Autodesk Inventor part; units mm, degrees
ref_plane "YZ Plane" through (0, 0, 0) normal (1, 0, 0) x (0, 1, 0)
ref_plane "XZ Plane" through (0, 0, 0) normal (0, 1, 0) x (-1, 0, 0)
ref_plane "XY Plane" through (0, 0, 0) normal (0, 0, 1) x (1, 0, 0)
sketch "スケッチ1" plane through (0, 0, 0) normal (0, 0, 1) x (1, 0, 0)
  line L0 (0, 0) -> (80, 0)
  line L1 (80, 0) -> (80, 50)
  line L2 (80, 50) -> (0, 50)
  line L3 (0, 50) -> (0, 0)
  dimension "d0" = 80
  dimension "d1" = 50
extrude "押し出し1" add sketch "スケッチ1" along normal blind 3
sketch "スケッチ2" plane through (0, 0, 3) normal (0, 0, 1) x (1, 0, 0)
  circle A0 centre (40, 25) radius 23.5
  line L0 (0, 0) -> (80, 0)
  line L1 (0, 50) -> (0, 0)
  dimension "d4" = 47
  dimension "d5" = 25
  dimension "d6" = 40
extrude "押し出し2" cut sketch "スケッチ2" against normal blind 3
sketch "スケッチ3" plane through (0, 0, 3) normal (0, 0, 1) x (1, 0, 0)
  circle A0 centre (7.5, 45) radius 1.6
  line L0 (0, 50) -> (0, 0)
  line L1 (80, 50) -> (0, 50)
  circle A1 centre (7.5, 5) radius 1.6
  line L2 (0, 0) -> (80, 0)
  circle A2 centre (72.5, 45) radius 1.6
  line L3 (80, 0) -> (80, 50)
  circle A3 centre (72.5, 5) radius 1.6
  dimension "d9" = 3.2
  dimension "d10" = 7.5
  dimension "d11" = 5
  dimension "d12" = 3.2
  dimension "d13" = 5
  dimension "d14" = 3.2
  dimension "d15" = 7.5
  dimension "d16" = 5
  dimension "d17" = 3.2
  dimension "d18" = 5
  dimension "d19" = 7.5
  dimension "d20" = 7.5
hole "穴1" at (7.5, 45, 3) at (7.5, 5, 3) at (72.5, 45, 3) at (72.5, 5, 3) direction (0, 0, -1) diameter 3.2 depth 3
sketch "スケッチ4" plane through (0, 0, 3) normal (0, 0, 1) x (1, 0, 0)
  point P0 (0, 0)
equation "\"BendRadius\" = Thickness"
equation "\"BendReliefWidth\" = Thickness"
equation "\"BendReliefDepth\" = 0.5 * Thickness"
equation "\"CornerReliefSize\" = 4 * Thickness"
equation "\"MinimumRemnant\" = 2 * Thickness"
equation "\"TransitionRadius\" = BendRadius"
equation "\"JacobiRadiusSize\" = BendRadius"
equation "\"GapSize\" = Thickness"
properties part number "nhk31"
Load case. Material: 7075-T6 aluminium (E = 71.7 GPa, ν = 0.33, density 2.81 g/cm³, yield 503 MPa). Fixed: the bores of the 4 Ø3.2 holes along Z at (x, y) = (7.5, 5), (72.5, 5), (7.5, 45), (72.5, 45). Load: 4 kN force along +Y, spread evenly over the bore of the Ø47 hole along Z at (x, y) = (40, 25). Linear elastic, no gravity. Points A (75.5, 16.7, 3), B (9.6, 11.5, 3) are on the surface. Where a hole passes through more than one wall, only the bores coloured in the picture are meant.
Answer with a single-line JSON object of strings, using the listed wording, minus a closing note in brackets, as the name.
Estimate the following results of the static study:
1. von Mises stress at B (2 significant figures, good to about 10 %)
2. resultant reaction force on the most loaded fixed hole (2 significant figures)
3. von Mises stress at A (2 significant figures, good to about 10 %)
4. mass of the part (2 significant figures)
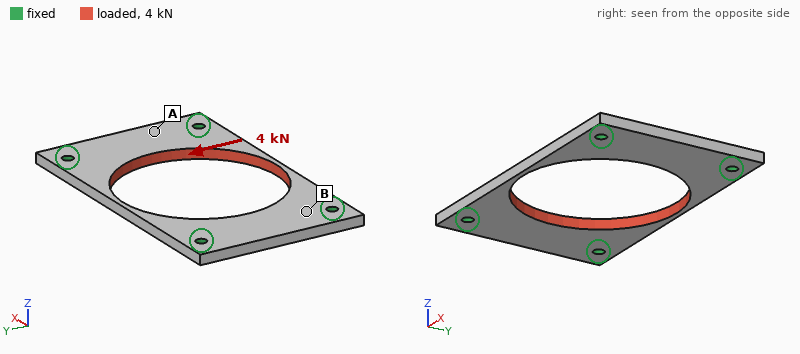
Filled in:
{"von Mises stress at B": "34 MPa", "resultant reaction force on the most loaded fixed hole": "1.0 kN", "von Mises stress at A": "20 MPa", "mass of the part": "19 g"}
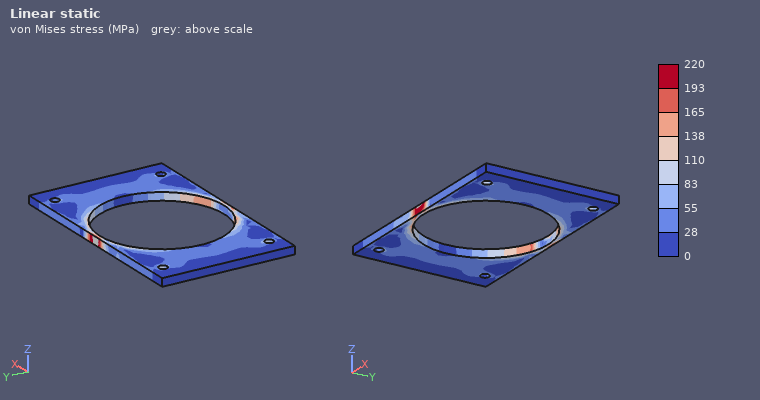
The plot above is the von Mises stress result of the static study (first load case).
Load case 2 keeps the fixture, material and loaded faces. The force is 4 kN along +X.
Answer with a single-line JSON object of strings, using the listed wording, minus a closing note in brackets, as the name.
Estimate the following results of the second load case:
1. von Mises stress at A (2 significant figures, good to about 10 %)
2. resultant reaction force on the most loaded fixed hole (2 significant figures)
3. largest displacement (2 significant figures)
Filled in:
{"von Mises stress at A": "10 MPa", "resultant reaction force on the most loaded fixed hole": "1.0 kN", "largest displacement": "11 µm"}
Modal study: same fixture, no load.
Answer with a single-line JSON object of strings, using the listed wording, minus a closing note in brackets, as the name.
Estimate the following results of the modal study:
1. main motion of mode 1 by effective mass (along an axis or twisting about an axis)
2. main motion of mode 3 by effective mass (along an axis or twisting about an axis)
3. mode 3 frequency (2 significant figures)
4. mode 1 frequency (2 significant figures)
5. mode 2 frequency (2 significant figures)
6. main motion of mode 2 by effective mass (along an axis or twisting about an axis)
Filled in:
{"main motion of mode 1 by effective mass": "along Z", "main motion of mode 3 by effective mass": "twisting about Y", "mode 3 frequency": "8800 Hz", "mode 1 frequency": "5600 Hz", "mode 2 frequency": "5800 Hz", "main motion of mode 2 by effective mass": "twisting about X"}
